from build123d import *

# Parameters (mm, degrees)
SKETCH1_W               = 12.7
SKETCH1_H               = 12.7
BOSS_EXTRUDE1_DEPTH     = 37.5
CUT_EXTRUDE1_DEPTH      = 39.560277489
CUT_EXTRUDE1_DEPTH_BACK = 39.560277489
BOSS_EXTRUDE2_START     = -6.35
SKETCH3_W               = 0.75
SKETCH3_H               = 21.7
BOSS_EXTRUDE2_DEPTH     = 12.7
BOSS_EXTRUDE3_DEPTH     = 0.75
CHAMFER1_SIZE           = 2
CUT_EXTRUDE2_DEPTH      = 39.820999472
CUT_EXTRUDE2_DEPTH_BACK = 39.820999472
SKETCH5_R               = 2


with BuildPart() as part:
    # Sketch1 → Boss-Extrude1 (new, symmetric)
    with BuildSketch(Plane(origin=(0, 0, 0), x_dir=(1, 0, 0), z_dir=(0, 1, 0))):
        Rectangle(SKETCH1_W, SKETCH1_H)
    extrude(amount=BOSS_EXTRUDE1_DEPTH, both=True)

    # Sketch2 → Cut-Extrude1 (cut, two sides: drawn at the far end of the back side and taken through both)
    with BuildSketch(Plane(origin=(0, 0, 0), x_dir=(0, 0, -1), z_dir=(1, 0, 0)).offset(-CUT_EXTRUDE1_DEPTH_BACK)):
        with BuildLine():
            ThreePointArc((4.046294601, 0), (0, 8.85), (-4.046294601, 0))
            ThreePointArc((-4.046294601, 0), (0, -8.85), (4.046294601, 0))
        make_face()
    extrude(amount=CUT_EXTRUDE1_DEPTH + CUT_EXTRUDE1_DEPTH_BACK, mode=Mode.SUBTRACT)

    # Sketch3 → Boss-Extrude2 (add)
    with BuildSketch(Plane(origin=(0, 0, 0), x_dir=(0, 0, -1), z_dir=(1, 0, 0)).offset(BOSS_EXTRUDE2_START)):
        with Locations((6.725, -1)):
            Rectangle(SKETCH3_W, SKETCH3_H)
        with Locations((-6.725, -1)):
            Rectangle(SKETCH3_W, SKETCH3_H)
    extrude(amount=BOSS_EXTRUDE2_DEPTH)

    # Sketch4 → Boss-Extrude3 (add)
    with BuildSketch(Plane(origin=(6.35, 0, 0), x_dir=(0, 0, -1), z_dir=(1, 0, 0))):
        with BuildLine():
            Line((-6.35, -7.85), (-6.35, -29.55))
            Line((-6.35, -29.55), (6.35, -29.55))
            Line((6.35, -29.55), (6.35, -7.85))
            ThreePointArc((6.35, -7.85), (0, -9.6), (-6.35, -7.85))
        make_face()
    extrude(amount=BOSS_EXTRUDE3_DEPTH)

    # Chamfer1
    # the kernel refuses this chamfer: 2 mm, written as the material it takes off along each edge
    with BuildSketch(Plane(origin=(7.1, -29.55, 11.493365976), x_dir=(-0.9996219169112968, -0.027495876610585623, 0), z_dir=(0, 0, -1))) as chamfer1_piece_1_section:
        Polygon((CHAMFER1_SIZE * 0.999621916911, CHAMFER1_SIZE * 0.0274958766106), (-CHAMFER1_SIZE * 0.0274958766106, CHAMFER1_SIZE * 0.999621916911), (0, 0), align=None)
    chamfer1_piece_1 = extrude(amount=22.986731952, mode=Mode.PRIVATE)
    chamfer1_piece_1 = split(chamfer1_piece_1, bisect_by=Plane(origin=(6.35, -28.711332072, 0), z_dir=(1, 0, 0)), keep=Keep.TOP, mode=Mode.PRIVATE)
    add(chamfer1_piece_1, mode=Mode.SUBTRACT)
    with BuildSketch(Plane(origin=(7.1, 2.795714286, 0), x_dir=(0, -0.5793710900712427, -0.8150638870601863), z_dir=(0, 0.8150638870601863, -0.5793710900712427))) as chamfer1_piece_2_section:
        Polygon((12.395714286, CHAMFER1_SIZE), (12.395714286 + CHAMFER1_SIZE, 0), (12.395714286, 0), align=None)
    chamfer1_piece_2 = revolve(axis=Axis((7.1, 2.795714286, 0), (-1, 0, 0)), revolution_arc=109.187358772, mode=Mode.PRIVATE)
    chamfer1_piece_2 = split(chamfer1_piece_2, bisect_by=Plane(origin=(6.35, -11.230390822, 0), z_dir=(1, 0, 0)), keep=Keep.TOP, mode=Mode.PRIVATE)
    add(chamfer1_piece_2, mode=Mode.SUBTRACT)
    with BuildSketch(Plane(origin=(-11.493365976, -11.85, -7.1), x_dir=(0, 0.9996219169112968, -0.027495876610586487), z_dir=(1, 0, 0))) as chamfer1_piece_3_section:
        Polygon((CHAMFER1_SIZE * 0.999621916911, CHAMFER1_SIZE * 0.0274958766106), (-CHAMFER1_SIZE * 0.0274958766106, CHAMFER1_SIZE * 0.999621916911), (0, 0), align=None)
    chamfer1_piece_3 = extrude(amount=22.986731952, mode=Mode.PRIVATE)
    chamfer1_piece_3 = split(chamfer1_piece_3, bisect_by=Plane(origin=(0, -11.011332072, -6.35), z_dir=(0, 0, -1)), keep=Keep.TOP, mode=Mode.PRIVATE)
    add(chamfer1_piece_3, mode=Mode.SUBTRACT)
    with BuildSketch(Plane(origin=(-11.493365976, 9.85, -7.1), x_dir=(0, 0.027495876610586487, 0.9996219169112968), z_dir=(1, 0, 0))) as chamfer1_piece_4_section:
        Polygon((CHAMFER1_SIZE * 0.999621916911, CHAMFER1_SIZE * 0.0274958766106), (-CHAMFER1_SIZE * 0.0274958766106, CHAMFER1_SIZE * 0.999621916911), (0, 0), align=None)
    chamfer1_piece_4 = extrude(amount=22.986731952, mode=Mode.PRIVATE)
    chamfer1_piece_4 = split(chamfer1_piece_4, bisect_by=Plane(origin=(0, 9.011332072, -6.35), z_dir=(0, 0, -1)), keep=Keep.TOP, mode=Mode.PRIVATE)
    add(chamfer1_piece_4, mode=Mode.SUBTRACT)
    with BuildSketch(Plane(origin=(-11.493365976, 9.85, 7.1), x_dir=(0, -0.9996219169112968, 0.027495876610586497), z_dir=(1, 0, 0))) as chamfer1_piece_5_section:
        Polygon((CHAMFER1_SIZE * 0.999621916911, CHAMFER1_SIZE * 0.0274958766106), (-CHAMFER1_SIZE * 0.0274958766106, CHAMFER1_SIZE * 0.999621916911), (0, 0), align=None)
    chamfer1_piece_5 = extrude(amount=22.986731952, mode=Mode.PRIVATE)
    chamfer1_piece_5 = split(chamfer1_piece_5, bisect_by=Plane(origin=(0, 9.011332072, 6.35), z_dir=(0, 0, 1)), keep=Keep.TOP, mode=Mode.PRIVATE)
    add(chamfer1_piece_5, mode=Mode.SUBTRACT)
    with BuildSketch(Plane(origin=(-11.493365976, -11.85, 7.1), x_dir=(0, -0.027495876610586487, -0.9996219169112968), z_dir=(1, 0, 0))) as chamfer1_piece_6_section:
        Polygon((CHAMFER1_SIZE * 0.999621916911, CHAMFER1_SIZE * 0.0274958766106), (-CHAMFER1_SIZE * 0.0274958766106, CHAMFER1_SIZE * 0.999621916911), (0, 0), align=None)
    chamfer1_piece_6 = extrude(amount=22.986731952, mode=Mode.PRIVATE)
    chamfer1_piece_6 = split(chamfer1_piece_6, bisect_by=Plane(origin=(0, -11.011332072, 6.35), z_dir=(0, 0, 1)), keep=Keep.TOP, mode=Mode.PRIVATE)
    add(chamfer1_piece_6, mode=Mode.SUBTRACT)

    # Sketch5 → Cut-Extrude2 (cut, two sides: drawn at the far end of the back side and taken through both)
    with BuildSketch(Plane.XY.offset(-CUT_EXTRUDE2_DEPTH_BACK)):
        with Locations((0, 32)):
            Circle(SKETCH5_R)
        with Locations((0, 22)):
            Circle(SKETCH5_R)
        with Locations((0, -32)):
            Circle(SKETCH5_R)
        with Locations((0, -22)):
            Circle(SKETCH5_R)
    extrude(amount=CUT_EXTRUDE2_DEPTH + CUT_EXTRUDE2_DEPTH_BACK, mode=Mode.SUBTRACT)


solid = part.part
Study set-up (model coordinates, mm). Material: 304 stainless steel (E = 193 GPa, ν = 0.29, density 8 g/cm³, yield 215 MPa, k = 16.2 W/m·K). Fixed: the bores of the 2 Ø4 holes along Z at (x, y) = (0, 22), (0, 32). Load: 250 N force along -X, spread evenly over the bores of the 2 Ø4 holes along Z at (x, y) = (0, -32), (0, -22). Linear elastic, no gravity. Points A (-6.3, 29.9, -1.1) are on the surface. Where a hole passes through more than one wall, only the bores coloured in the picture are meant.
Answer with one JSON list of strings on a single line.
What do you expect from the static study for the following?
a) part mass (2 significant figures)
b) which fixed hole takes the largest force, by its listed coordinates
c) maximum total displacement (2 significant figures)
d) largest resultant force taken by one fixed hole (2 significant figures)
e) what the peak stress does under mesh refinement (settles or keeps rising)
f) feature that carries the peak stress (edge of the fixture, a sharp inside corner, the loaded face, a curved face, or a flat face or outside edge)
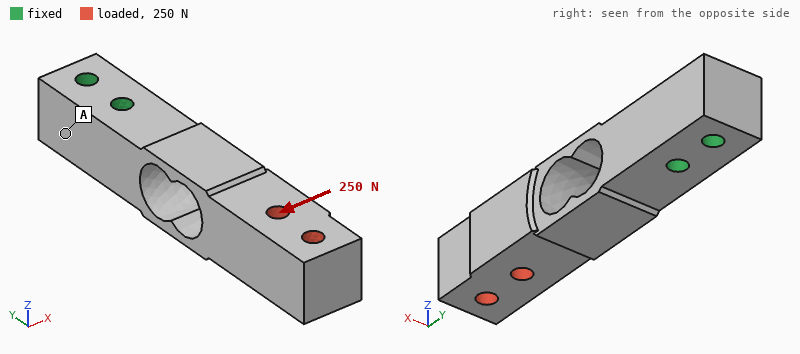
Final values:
["80 g", "(0, 22)", "73 µm", "810 N", "keeps rising", "a sharp inside corner"]
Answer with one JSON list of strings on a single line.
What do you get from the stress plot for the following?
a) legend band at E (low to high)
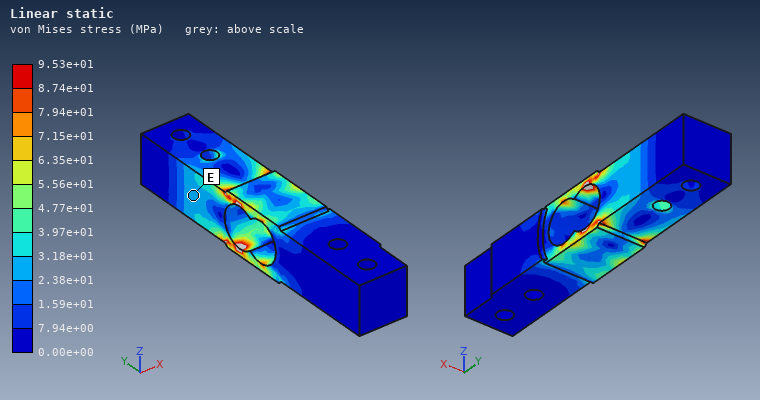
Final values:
["2.38e+01 to 3.18e+01 MPa"]
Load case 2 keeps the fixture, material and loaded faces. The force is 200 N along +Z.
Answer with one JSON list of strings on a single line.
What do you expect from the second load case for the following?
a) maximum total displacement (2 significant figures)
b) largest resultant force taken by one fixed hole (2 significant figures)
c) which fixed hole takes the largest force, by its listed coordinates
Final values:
["49 µm", "310 N", "(0, 22)"]
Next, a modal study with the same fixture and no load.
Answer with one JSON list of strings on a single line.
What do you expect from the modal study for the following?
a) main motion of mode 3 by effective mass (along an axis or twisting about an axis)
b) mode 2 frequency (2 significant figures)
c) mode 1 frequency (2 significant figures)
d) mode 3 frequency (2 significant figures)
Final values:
["twisting about Y", "1900 Hz", "1900 Hz", "7700 Hz"]
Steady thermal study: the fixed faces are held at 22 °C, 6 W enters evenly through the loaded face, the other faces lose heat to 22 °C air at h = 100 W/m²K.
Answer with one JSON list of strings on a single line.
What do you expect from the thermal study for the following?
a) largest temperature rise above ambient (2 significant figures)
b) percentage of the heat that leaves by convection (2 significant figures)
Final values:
["35 K", "94 %"]
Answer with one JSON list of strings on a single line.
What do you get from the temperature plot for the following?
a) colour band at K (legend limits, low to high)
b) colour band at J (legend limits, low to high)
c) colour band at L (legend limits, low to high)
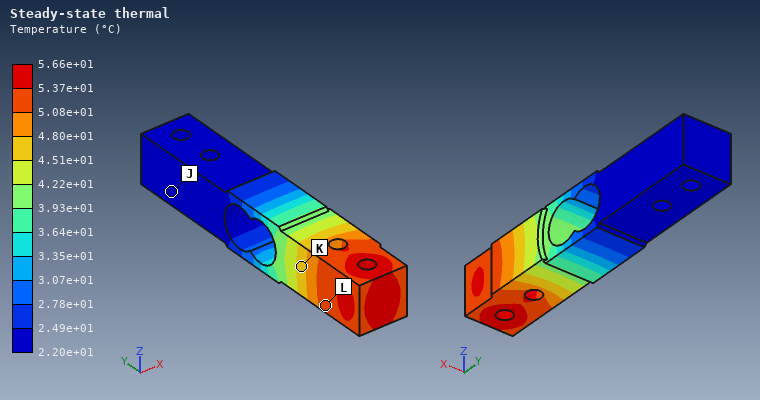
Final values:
["4.51e+01 to 4.80e+01 °C", "2.20e+01 to 2.49e+01 °C", "5.08e+01 to 5.37e+01 °C"]
